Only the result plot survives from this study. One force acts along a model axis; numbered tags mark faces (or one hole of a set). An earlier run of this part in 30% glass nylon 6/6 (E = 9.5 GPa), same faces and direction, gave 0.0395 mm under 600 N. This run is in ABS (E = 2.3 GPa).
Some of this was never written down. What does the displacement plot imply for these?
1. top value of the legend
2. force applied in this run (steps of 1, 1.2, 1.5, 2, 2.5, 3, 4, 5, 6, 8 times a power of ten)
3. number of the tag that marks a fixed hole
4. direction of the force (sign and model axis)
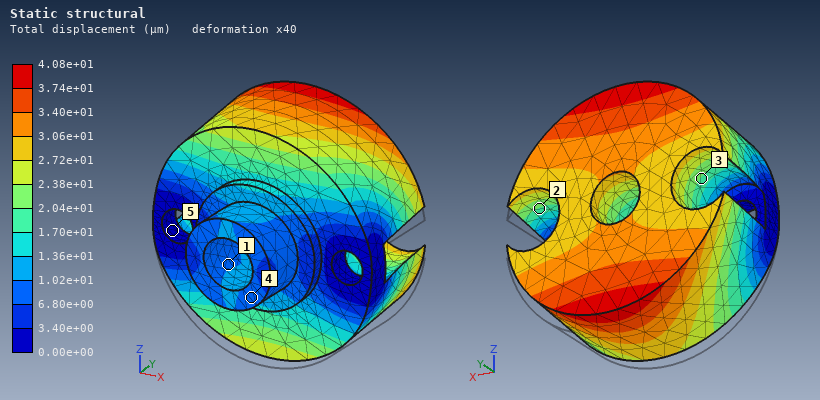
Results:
4.08e+01 µm
150 N
5
+Z
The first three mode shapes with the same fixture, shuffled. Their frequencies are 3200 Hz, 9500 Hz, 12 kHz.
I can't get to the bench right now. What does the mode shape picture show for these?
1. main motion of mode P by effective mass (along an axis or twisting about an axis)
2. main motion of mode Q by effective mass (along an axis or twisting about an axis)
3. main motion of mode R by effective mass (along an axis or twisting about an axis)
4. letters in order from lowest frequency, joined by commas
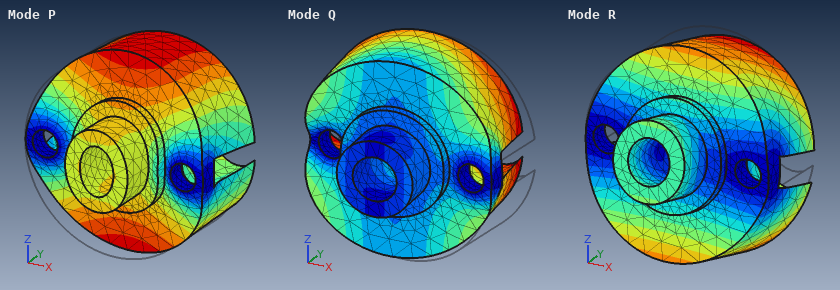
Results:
along Y
along X
along Z
R, P, Q
